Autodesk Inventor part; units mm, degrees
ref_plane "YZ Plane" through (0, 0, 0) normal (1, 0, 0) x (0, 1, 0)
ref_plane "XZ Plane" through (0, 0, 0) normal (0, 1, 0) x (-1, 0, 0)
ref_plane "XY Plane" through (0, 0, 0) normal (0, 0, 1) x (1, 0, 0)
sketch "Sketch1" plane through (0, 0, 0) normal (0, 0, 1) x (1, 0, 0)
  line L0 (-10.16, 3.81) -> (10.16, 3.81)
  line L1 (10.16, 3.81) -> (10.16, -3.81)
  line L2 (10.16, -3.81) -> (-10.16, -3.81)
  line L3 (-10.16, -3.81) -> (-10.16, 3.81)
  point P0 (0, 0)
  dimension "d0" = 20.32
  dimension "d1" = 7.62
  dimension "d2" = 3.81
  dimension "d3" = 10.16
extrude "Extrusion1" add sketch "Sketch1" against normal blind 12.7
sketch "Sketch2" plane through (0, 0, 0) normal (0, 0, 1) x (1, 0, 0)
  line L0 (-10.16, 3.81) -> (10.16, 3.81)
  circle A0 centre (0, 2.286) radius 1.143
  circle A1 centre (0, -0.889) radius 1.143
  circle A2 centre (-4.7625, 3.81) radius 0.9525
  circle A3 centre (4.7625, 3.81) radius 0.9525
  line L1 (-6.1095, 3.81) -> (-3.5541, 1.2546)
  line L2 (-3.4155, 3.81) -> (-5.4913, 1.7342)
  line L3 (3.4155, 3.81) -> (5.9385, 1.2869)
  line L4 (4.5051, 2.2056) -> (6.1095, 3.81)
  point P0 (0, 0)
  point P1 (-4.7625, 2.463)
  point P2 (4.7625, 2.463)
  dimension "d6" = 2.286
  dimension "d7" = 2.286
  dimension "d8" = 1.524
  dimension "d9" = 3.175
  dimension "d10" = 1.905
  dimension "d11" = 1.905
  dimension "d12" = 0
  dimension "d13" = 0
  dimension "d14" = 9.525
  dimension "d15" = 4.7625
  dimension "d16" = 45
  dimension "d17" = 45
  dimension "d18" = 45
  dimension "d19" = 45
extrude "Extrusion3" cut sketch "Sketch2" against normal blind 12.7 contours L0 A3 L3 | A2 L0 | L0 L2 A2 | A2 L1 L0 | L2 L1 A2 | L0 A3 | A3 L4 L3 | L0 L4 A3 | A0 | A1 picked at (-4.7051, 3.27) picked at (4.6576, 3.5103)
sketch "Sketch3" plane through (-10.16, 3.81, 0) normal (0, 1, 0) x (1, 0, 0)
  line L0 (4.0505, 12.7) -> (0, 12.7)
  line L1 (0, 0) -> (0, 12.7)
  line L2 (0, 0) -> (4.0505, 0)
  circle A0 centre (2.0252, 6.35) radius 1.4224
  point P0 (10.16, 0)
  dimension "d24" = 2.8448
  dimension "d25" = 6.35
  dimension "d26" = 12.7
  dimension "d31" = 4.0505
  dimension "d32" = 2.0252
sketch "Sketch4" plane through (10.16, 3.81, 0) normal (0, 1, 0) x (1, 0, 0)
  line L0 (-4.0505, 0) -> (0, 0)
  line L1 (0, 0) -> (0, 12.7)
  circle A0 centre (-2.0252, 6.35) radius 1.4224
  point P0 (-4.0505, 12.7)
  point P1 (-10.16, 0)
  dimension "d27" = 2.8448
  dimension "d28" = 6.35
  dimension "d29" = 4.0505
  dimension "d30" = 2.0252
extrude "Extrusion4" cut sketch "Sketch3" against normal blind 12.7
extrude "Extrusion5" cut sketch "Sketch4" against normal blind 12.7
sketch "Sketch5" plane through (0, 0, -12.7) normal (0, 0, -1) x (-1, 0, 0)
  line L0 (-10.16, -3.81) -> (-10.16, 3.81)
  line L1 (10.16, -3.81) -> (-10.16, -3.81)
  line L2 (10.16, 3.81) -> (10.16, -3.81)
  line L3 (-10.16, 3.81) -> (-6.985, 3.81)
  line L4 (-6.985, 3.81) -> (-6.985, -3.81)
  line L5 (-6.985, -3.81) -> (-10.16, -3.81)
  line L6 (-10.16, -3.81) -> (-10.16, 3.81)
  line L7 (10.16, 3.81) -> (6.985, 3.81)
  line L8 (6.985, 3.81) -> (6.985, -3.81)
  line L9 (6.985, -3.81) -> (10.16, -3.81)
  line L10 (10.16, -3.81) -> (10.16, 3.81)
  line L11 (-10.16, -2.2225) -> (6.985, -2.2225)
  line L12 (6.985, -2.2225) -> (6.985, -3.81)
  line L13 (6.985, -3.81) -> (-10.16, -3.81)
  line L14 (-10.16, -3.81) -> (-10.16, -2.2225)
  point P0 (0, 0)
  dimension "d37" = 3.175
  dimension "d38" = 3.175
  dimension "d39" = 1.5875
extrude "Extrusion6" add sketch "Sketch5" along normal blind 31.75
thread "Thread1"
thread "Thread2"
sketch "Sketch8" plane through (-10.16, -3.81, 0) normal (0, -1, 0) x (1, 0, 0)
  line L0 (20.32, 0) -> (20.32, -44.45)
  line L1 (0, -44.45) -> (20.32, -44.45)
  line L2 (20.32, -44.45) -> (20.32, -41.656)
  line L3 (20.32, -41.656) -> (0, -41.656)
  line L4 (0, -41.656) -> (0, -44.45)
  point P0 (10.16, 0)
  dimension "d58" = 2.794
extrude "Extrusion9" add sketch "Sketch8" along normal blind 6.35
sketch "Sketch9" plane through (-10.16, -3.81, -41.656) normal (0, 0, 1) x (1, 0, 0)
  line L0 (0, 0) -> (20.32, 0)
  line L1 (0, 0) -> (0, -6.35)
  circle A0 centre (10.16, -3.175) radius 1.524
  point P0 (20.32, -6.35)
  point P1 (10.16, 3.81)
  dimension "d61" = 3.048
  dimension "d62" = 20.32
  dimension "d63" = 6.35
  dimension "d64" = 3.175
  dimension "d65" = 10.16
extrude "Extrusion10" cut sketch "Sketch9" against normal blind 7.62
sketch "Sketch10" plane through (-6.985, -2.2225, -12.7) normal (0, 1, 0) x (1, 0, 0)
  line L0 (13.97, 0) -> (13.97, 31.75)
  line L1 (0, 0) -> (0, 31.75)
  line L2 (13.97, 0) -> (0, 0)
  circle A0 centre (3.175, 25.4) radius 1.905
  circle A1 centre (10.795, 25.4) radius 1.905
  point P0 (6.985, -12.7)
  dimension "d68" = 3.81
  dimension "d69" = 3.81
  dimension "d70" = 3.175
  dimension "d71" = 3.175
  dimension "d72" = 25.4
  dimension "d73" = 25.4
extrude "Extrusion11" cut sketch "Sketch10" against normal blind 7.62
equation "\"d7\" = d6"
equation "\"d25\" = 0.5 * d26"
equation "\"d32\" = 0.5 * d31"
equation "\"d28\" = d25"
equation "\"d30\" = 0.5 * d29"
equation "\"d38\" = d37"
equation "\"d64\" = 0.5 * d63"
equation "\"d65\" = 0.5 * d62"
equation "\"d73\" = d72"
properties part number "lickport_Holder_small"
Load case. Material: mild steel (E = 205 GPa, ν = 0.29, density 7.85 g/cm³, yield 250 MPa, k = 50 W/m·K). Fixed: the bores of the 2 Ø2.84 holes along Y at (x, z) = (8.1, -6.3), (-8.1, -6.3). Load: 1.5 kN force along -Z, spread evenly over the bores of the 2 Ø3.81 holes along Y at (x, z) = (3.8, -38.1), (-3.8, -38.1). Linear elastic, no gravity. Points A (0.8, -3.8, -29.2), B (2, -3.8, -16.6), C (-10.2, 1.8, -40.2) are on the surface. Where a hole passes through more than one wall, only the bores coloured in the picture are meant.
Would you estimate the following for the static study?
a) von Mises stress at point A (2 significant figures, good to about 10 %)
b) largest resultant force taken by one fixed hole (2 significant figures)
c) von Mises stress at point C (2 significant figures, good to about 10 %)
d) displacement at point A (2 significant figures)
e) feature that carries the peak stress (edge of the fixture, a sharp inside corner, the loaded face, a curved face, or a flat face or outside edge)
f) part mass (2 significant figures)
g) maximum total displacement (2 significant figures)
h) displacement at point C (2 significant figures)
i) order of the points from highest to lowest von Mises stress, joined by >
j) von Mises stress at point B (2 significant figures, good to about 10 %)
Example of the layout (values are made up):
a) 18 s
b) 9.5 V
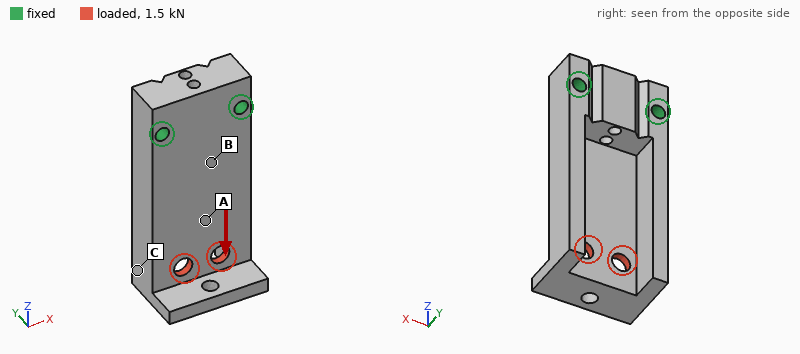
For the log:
a) 55 MPa
b) 750 N
c) 6.8 MPa
d) 12 µm
e) the loaded face
f) 33 g
g) 31 µm
h) 21 µm
i) A > B > C
j) 41 MPa
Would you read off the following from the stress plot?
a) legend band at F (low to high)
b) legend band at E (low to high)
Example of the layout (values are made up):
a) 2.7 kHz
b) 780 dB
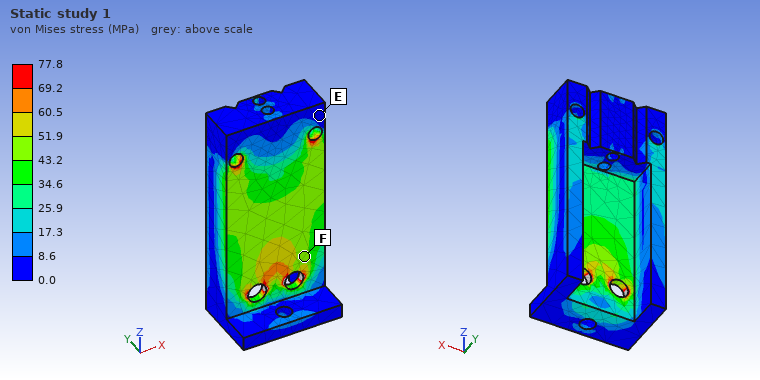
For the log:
a) 43.2 to 51.9 MPa
b) 0.0 to 8.6 MPa
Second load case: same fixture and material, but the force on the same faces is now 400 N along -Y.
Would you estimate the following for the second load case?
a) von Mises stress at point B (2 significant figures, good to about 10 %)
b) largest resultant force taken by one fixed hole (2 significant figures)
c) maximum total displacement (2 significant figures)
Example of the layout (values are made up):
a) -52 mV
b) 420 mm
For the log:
a) 56 MPa
b) 240 N
c) 72 µm
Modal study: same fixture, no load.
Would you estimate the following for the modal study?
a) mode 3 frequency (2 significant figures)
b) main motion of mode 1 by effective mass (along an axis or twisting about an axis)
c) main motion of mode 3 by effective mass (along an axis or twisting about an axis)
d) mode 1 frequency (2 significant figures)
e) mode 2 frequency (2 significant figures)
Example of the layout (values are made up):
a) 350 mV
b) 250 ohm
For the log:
a) 9500 Hz
b) along Y
c) along X
d) 3800 Hz
e) 5400 Hz
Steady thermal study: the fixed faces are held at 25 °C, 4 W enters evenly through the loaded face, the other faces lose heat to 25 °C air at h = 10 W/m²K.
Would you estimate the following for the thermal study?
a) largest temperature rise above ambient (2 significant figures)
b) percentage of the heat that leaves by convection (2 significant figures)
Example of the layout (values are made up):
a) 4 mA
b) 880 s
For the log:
a) 37 K
b) 13 %
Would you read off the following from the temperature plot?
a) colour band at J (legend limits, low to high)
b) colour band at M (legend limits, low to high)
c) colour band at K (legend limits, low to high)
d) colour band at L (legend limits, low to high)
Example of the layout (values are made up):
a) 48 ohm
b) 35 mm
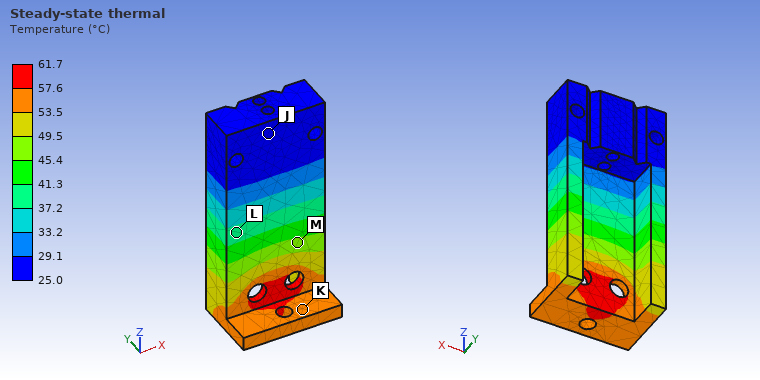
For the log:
a) 25.0 to 29.1 °C
b) 45.4 to 49.5 °C
c) 53.5 to 57.6 °C
d) 37.2 to 41.3 °C
